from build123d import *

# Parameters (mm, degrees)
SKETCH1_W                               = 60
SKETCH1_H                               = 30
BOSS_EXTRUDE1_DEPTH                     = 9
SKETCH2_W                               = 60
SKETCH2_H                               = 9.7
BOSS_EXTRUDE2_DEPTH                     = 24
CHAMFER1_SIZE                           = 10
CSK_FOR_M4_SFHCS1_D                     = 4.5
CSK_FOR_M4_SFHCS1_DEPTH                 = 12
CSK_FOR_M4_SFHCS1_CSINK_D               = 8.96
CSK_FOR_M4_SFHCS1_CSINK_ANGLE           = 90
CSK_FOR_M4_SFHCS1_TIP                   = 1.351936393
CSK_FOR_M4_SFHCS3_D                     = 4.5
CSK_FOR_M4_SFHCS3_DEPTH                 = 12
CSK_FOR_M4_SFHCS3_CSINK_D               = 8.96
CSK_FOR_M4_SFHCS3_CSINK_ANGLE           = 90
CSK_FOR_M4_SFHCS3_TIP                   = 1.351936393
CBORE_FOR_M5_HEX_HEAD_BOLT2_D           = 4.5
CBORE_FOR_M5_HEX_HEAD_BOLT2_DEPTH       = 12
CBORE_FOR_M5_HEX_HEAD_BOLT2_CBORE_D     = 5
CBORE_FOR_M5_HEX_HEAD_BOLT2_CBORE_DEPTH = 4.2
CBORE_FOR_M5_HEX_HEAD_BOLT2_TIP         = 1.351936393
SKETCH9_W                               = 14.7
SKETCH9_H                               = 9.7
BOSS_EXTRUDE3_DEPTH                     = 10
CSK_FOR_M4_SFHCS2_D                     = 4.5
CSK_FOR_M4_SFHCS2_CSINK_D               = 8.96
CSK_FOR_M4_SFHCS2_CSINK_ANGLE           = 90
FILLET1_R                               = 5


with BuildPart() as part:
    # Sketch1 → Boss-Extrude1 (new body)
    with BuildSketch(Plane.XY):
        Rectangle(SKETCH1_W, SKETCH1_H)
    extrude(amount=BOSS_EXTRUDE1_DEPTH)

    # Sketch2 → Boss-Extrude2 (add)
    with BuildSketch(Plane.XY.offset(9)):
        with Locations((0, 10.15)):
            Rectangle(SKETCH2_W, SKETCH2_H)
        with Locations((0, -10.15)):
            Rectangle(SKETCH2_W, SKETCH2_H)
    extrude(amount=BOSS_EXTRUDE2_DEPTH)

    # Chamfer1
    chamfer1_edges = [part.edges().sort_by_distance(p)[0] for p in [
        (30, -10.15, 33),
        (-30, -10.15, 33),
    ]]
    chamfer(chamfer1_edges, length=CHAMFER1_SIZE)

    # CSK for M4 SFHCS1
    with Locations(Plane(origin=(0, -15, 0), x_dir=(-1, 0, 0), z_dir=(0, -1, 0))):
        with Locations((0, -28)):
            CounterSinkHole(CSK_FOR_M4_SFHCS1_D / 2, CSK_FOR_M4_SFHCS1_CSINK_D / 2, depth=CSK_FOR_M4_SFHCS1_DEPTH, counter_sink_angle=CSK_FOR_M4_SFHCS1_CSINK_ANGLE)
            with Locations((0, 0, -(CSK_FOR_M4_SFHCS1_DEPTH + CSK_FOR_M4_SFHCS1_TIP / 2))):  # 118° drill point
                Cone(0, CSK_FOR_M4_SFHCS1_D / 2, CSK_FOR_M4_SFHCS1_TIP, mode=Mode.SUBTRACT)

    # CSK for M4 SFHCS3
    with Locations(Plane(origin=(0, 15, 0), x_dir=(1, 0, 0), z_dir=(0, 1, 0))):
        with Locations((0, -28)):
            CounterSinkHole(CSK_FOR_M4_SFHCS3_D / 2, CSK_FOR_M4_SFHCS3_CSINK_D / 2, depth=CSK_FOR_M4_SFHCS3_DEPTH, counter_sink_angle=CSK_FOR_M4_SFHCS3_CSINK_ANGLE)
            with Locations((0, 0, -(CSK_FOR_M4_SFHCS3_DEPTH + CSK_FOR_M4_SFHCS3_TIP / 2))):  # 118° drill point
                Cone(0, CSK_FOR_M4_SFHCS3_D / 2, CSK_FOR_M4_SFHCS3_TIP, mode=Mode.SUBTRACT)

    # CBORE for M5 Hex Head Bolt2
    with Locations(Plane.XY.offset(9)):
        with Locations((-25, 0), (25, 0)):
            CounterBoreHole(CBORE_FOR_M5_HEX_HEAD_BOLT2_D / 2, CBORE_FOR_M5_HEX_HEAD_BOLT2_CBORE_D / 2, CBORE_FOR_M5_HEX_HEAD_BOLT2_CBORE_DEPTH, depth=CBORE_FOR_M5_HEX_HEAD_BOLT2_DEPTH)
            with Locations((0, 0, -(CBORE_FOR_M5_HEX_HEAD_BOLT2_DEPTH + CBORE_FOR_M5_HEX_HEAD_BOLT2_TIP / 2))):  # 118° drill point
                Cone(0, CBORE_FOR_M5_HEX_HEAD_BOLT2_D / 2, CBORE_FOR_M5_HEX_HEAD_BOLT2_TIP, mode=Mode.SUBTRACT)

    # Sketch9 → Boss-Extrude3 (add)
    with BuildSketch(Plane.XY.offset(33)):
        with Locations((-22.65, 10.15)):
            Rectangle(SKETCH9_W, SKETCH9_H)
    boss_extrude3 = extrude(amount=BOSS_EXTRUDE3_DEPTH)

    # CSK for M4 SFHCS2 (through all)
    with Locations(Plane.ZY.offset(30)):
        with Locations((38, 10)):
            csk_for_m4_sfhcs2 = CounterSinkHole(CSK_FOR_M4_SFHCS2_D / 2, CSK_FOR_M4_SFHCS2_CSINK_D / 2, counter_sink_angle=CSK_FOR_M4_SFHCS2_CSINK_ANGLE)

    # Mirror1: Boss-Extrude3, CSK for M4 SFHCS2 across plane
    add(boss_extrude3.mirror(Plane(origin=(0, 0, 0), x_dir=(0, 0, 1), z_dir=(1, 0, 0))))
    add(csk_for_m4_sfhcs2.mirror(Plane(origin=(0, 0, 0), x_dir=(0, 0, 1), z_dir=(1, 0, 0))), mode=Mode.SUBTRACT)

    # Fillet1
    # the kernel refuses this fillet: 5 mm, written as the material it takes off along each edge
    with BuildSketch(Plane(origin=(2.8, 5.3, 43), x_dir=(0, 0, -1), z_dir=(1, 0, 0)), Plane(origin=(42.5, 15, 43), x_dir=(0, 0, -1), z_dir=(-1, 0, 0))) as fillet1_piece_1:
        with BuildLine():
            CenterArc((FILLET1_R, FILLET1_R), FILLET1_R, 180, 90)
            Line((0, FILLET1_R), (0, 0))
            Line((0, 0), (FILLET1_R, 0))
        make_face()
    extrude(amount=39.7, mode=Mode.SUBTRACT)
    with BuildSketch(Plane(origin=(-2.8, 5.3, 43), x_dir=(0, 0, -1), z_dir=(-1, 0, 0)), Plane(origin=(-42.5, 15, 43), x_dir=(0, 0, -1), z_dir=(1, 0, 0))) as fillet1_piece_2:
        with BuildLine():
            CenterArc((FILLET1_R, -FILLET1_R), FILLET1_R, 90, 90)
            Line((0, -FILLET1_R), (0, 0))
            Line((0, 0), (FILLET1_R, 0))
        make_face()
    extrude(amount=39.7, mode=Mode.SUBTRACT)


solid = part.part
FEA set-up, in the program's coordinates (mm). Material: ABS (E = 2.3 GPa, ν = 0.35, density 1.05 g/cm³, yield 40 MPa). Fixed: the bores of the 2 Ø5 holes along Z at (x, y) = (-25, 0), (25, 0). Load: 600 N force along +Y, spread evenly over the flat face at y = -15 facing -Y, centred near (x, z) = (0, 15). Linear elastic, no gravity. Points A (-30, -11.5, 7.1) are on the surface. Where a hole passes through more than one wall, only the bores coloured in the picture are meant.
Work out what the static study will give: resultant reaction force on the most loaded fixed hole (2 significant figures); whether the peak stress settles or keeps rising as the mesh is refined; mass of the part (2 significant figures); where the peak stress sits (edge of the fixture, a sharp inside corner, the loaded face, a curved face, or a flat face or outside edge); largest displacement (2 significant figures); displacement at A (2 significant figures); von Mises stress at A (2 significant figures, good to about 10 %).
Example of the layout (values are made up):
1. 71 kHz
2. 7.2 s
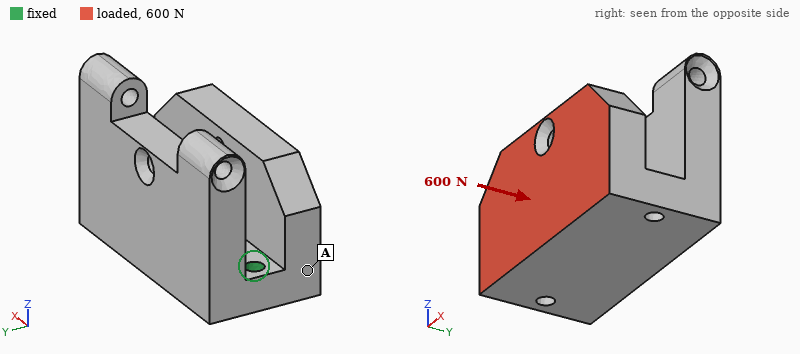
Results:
1. 300 N
2. keeps rising
3. 47 g
4. edge of the fixture
5. 0.60 mm
6. 0.14 mm
7. 4.2 MPa
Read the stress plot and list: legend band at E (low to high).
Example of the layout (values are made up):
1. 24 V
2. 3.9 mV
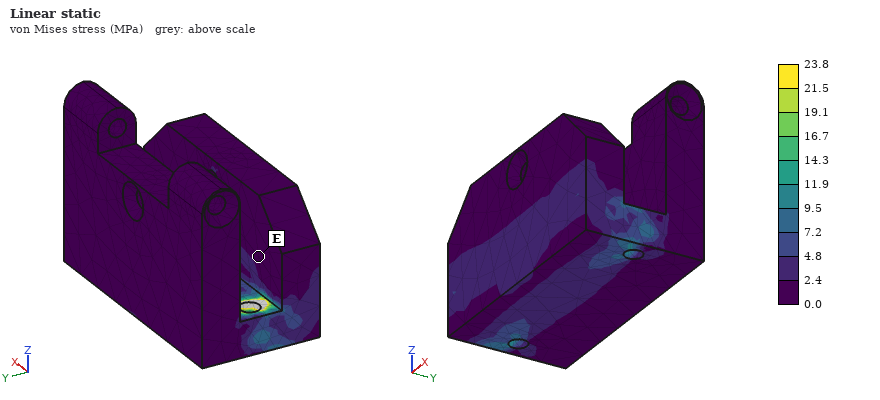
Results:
1. 0.0 to 2.4 MPa
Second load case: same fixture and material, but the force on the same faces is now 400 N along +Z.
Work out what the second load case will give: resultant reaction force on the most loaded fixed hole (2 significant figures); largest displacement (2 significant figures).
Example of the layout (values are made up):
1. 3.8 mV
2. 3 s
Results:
1. 200 N
2. 0.50 mm
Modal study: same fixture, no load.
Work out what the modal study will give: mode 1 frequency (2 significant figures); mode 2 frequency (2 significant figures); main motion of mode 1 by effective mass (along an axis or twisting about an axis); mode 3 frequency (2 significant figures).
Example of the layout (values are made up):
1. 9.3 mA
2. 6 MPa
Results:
1. 870 Hz
2. 1800 Hz
3. along Y
4. 2100 Hz
